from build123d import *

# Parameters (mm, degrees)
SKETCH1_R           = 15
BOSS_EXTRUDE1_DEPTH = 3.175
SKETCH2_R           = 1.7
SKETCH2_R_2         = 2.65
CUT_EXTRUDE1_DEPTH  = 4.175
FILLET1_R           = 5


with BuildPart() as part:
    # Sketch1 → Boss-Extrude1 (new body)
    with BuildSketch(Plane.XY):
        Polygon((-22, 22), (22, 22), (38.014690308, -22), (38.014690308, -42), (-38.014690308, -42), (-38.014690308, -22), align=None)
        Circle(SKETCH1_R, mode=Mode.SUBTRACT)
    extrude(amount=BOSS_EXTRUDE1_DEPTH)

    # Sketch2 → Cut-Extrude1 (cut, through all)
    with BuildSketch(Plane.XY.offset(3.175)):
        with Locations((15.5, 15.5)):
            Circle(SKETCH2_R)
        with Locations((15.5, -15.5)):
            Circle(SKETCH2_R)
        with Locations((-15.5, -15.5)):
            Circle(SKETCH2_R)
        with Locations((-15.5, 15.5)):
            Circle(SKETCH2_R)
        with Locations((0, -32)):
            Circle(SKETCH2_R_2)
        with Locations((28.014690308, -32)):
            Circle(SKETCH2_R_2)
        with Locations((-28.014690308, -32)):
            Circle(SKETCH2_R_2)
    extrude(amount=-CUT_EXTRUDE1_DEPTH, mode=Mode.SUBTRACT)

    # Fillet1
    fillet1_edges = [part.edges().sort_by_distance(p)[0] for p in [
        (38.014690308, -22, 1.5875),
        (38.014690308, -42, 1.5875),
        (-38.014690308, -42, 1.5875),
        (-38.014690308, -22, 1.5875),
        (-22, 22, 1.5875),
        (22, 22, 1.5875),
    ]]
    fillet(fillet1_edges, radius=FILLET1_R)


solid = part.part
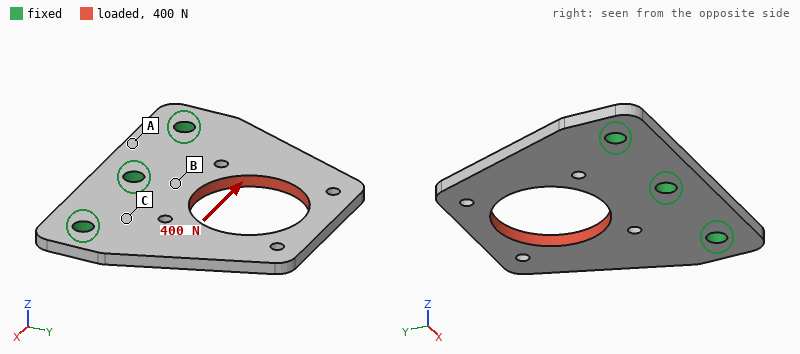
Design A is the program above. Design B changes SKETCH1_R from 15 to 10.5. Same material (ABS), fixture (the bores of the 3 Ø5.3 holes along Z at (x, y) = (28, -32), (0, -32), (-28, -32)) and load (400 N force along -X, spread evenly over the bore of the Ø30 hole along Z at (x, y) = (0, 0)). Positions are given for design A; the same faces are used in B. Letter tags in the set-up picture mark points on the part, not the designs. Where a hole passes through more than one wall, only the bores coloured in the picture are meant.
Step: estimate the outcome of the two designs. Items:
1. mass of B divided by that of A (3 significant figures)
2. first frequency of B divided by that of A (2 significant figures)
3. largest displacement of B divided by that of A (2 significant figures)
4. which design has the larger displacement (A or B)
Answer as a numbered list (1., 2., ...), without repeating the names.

1. 1.11
2. 0.99
3. 0.60
4. A
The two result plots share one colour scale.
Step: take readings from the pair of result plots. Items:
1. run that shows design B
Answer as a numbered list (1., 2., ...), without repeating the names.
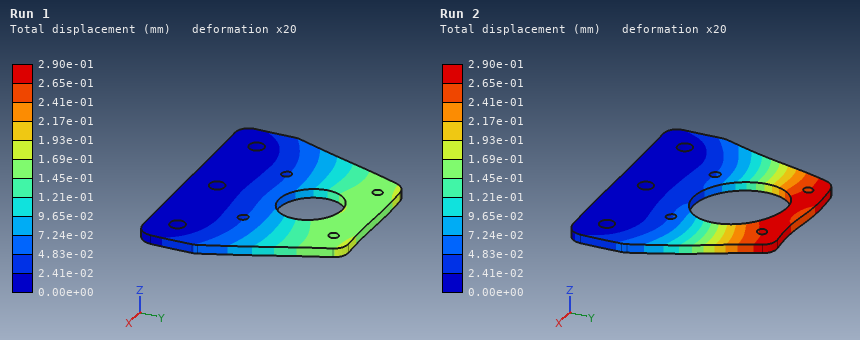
1. Run 1
